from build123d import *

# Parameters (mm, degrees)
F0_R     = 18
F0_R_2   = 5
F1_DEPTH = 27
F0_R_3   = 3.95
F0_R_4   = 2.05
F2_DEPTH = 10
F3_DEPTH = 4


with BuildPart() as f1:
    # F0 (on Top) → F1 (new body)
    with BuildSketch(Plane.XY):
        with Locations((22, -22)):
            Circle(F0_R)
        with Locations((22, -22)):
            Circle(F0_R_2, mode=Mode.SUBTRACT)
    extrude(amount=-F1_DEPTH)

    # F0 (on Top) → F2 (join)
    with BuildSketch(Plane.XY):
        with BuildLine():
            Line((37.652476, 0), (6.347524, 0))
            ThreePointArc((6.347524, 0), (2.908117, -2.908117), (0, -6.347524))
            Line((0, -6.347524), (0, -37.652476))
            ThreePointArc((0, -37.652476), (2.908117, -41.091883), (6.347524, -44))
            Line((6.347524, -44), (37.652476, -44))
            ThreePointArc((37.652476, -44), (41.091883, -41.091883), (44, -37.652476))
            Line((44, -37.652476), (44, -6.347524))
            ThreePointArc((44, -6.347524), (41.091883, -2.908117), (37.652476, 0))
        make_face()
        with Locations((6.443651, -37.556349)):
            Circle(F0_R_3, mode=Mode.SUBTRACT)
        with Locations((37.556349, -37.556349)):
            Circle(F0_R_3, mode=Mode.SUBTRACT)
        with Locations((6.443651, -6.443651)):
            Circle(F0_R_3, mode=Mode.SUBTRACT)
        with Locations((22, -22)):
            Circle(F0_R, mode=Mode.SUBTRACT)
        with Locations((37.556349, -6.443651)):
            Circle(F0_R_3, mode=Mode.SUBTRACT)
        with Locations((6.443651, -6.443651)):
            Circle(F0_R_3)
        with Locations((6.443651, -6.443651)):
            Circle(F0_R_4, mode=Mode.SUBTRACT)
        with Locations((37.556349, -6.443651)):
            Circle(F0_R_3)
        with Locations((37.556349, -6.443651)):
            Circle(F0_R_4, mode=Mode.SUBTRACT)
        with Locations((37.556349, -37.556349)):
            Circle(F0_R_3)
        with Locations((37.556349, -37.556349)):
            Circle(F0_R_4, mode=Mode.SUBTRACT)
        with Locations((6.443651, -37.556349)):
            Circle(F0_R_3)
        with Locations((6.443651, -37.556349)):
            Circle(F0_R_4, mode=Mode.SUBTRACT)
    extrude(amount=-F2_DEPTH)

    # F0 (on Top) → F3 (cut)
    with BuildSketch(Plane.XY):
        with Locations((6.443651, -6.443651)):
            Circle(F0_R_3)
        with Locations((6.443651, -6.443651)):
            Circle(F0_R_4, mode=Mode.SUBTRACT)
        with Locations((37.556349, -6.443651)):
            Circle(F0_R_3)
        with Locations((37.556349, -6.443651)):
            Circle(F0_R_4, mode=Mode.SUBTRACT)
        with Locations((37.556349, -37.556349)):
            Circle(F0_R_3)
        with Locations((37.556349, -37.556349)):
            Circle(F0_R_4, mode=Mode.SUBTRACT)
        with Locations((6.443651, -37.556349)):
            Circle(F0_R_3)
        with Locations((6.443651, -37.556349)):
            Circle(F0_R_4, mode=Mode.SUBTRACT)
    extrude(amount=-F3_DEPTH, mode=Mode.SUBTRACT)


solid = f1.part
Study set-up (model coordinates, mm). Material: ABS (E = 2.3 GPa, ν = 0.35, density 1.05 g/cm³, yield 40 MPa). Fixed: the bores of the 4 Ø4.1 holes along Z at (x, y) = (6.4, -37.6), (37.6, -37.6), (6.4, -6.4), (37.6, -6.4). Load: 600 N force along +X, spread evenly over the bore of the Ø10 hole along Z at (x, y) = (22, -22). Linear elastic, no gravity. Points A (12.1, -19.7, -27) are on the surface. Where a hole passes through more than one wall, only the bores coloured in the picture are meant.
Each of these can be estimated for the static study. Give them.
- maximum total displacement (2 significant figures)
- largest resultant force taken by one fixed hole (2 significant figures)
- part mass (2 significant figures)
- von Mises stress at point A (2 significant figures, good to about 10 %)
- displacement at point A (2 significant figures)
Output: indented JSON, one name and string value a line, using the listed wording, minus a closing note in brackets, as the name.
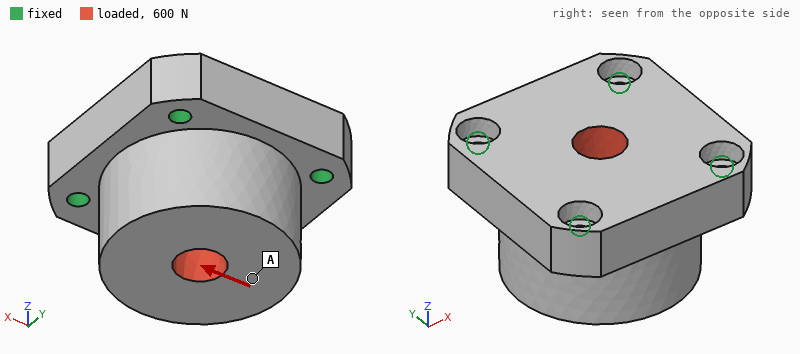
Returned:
{
  "maximum total displacement": "27 µm",
  "largest resultant force taken by one fixed hole": "170 N",
  "part mass": "34 g",
  "von Mises stress at point A": "0.62 MPa",
  "displacement at point A": "25 µm"
}
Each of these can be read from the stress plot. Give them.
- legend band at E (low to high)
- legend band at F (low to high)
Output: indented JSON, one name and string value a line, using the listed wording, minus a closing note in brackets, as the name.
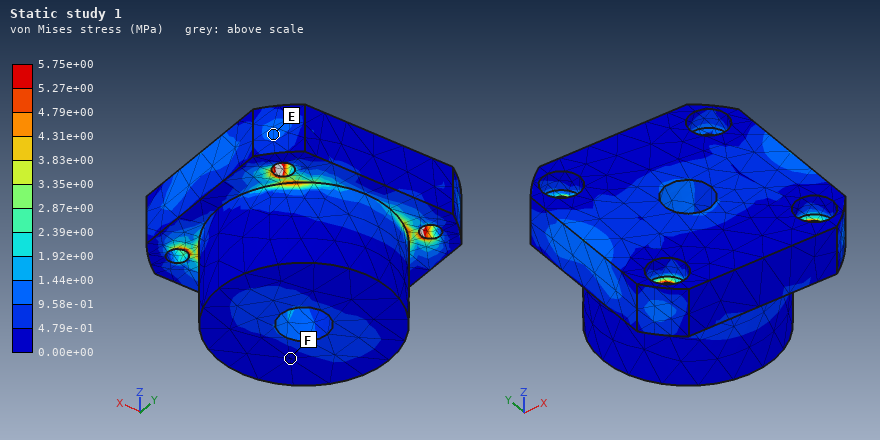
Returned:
{
  "legend band at E": "9.58e-01 to 1.44e+00 MPa",
  "legend band at F": "0.00e+00 to 4.79e-01 MPa"
}
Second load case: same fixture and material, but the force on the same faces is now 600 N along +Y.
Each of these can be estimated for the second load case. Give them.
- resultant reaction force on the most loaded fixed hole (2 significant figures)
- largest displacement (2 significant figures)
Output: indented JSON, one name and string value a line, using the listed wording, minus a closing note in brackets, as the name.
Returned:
{
  "resultant reaction force on the most loaded fixed hole": "170 N",
  "largest displacement": "27 µm"
}
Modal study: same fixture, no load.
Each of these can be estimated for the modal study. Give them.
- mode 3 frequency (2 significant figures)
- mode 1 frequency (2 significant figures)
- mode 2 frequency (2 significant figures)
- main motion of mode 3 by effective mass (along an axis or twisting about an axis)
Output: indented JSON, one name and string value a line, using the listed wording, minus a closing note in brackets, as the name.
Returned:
{
  "mode 3 frequency": "5600 Hz",
  "mode 1 frequency": "5300 Hz",
  "mode 2 frequency": "5300 Hz",
  "main motion of mode 3 by effective mass": "along Z"
}
